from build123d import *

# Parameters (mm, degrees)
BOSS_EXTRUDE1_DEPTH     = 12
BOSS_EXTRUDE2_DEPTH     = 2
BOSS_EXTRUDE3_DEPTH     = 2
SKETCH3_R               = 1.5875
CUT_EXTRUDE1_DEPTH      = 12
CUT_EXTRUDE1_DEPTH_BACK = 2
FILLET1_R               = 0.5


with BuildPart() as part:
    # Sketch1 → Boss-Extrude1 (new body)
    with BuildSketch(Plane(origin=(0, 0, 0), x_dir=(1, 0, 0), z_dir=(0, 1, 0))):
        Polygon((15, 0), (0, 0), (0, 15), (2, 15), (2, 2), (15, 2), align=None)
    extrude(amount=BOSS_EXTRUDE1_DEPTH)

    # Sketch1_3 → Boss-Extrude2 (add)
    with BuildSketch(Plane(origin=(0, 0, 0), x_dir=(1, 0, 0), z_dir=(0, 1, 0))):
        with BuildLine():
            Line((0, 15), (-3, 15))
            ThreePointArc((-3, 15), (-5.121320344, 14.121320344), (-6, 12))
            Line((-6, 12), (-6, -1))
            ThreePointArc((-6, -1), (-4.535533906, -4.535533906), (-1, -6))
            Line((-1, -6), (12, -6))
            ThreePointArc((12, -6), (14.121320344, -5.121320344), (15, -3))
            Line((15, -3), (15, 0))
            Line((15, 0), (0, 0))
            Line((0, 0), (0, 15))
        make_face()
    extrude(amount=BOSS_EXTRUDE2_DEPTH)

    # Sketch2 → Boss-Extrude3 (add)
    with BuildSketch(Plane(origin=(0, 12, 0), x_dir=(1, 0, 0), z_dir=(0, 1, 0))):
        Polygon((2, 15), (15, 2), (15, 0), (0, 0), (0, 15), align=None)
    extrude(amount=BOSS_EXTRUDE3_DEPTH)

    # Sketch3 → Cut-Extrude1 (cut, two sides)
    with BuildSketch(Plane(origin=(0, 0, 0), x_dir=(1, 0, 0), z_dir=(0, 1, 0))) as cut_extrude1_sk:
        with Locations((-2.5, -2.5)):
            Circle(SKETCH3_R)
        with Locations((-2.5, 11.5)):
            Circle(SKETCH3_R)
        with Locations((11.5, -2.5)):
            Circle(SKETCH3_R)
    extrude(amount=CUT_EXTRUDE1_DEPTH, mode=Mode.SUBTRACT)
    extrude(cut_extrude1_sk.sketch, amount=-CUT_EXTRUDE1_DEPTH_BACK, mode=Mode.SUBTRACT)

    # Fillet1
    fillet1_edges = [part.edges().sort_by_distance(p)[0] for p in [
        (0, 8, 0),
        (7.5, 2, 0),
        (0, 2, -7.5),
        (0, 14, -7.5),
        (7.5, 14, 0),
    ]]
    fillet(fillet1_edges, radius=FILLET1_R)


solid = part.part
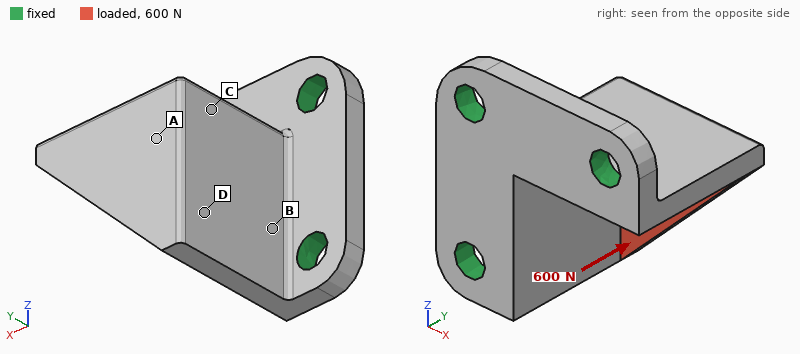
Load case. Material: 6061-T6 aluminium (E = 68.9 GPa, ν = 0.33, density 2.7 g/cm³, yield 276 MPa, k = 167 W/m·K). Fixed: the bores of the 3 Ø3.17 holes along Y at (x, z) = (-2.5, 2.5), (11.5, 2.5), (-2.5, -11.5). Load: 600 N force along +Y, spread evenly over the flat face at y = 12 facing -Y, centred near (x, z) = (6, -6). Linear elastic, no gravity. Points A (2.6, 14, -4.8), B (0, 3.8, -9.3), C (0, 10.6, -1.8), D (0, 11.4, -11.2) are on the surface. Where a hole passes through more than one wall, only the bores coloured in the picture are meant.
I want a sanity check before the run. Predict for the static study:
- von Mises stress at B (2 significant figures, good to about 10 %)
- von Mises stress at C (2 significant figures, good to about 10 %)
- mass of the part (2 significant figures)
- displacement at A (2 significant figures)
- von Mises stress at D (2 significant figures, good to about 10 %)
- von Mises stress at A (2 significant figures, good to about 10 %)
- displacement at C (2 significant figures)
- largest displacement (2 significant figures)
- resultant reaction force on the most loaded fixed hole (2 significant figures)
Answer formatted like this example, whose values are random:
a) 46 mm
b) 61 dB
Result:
a) 33 MPa
b) 19 MPa
c) 3.6 g
d) 17 µm
e) 50 MPa
f) 60 MPa
g) 8.4 µm
h) 45 µm
i) 330 N
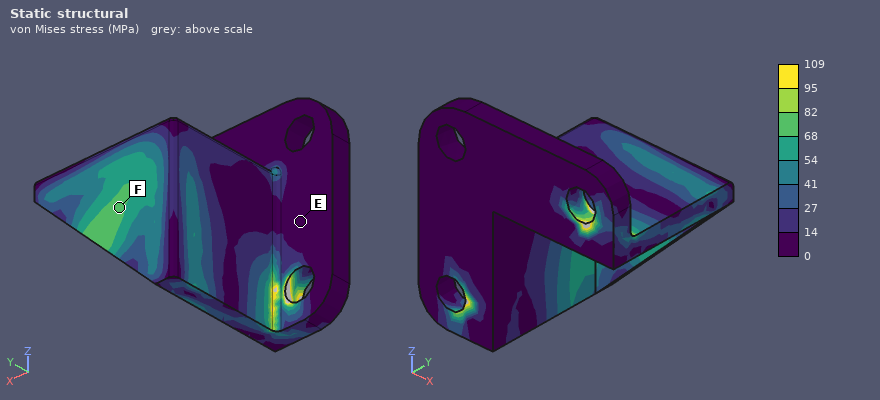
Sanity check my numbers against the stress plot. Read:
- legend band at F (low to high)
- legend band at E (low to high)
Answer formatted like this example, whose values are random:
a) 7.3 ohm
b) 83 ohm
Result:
a) 68 to 82 MPa
b) 0 to 14 MPa
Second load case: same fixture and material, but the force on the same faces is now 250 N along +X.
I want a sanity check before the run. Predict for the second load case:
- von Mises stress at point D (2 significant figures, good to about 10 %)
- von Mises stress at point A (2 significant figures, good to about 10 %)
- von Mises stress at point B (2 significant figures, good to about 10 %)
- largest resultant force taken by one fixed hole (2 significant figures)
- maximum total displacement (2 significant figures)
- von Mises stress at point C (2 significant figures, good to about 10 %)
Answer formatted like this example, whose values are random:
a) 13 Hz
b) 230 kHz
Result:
a) 33 MPa
b) 24 MPa
c) 34 MPa
d) 210 N
e) 51 µm
f) 23 MPa
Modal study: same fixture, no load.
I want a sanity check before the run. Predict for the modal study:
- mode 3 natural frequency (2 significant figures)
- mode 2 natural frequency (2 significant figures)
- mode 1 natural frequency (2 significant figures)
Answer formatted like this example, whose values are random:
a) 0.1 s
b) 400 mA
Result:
a) 27 kHz
b) 15 kHz
c) 12 kHz
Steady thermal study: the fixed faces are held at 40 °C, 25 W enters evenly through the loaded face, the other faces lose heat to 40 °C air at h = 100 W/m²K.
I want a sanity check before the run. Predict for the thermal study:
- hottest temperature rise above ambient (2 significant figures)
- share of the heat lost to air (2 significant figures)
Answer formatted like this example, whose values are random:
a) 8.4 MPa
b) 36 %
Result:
a) 49 K
b) 9.5 %
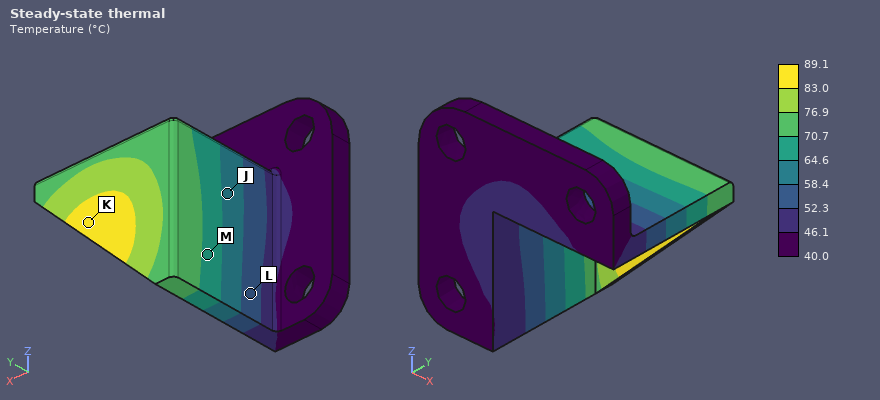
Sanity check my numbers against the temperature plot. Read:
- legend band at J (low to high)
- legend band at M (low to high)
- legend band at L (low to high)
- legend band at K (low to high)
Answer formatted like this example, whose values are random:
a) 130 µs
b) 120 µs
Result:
a) 58.4 to 64.6 °C
b) 64.6 to 70.7 °C
c) 52.3 to 58.4 °C
d) 83.0 to 89.1 °C
